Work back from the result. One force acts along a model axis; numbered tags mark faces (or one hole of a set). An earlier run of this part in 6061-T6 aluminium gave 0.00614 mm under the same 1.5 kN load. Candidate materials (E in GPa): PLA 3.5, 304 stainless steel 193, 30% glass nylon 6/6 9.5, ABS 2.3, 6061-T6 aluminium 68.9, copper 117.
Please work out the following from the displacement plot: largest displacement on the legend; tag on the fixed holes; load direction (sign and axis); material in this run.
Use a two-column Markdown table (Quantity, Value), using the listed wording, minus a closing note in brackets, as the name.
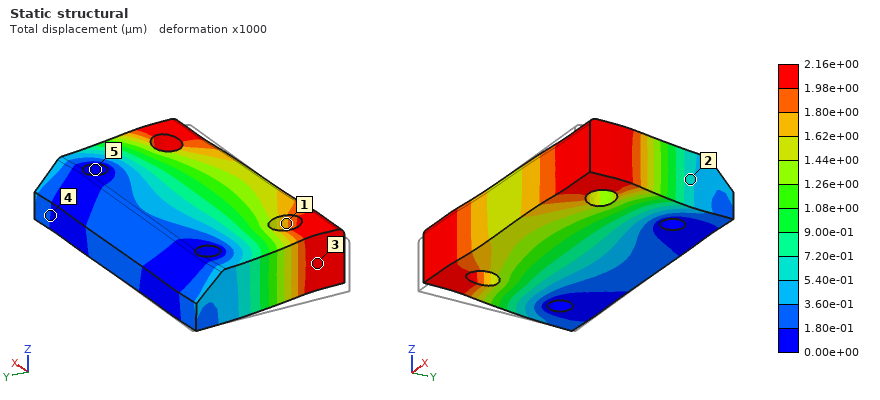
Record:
| Quantity | Value |
|---|---|
| largest displacement on the legend | 2.16e+00 µm |
| tag on the fixed holes | 5 |
| load direction | +X |
| material in this run | 304 stainless steel |
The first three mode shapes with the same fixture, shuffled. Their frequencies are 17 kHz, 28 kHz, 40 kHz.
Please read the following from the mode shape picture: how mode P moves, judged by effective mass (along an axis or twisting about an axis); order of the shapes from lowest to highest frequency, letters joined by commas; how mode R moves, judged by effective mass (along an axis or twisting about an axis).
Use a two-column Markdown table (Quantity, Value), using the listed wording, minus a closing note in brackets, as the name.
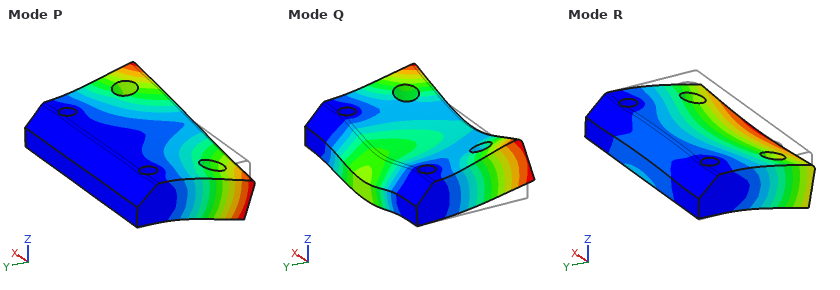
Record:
| Quantity | Value |
|---|---|
| how mode P moves, judged by effective mass | twisting about Y |
| order of the shapes from lowest to highest frequency, letters joined by commas | R, P, Q |
| how mode R moves, judged by effective mass | along Z |
